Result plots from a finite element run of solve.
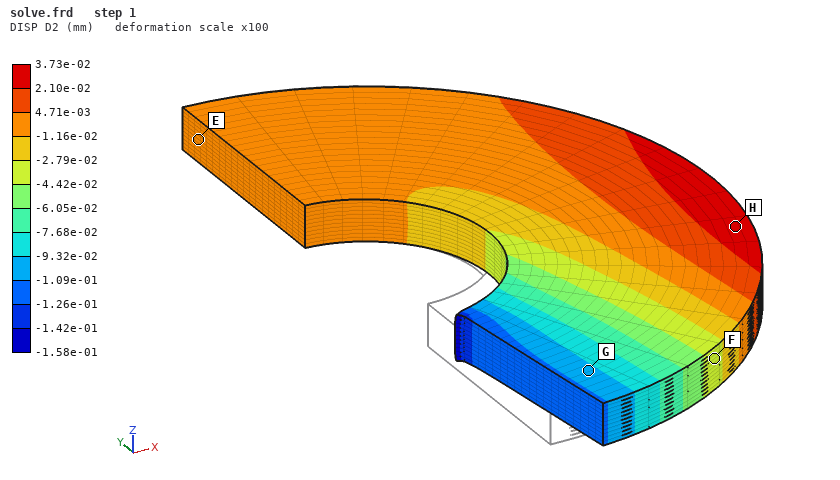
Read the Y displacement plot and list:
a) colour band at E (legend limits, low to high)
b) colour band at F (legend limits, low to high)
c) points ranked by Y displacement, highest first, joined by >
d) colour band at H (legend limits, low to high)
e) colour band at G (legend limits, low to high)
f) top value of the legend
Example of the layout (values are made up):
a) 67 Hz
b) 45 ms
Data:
a) -1.16e-02 to 4.71e-03 mm
b) -4.42e-02 to -2.79e-02 mm
c) H > E > F > G
d) 2.10e-02 to 3.73e-02 mm
e) -1.09e-01 to -9.32e-02 mm
f) 3.73e-02 mm
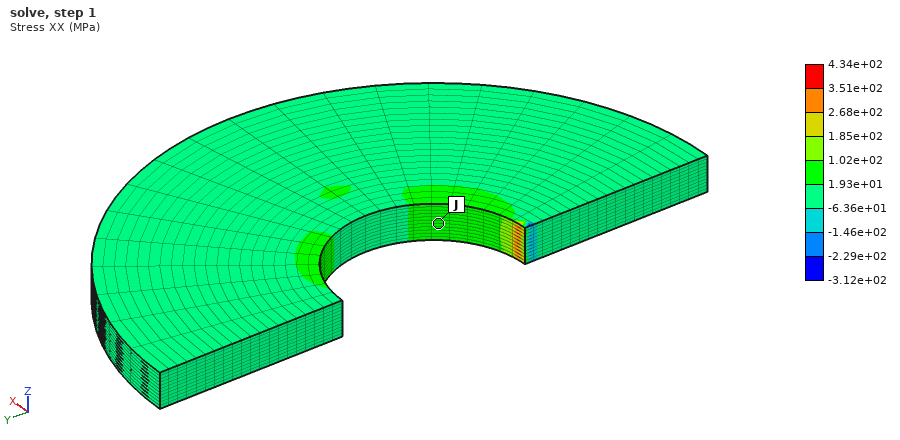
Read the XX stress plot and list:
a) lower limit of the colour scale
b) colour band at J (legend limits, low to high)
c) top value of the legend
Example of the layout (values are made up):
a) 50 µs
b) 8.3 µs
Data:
a) -3.12e+02 MPa
b) 1.93e+01 to 1.02e+02 MPa
c) 4.34e+02 MPa
